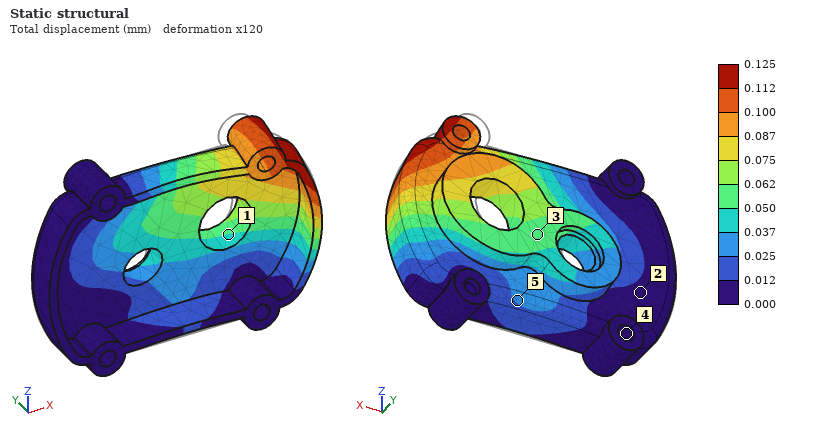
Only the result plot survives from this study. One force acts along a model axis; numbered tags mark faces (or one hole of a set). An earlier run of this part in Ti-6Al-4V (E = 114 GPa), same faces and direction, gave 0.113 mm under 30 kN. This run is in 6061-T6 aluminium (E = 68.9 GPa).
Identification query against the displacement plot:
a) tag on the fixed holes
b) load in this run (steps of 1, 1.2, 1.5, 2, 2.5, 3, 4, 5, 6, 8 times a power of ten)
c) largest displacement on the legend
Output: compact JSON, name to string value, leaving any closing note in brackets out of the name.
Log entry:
{"tag on the fixed holes": "4", "load in this run": "20 kN", "largest displacement on the legend": "0.125 mm"}
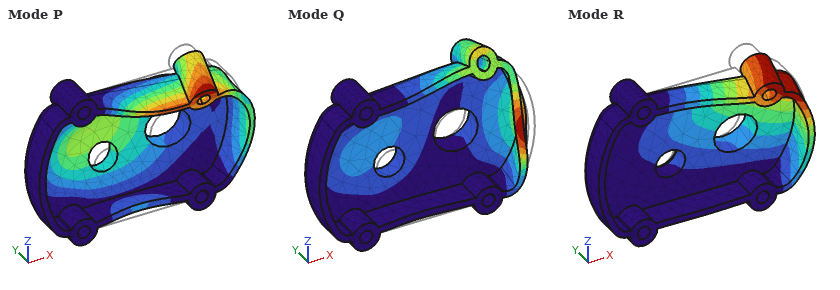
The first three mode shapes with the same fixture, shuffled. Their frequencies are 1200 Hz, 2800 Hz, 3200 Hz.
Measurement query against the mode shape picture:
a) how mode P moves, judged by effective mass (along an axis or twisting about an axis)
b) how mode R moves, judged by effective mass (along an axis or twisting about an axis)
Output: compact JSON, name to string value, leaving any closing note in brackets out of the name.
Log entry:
{"how mode P moves, judged by effective mass": "along Y", "how mode R moves, judged by effective mass": "along Y"}
